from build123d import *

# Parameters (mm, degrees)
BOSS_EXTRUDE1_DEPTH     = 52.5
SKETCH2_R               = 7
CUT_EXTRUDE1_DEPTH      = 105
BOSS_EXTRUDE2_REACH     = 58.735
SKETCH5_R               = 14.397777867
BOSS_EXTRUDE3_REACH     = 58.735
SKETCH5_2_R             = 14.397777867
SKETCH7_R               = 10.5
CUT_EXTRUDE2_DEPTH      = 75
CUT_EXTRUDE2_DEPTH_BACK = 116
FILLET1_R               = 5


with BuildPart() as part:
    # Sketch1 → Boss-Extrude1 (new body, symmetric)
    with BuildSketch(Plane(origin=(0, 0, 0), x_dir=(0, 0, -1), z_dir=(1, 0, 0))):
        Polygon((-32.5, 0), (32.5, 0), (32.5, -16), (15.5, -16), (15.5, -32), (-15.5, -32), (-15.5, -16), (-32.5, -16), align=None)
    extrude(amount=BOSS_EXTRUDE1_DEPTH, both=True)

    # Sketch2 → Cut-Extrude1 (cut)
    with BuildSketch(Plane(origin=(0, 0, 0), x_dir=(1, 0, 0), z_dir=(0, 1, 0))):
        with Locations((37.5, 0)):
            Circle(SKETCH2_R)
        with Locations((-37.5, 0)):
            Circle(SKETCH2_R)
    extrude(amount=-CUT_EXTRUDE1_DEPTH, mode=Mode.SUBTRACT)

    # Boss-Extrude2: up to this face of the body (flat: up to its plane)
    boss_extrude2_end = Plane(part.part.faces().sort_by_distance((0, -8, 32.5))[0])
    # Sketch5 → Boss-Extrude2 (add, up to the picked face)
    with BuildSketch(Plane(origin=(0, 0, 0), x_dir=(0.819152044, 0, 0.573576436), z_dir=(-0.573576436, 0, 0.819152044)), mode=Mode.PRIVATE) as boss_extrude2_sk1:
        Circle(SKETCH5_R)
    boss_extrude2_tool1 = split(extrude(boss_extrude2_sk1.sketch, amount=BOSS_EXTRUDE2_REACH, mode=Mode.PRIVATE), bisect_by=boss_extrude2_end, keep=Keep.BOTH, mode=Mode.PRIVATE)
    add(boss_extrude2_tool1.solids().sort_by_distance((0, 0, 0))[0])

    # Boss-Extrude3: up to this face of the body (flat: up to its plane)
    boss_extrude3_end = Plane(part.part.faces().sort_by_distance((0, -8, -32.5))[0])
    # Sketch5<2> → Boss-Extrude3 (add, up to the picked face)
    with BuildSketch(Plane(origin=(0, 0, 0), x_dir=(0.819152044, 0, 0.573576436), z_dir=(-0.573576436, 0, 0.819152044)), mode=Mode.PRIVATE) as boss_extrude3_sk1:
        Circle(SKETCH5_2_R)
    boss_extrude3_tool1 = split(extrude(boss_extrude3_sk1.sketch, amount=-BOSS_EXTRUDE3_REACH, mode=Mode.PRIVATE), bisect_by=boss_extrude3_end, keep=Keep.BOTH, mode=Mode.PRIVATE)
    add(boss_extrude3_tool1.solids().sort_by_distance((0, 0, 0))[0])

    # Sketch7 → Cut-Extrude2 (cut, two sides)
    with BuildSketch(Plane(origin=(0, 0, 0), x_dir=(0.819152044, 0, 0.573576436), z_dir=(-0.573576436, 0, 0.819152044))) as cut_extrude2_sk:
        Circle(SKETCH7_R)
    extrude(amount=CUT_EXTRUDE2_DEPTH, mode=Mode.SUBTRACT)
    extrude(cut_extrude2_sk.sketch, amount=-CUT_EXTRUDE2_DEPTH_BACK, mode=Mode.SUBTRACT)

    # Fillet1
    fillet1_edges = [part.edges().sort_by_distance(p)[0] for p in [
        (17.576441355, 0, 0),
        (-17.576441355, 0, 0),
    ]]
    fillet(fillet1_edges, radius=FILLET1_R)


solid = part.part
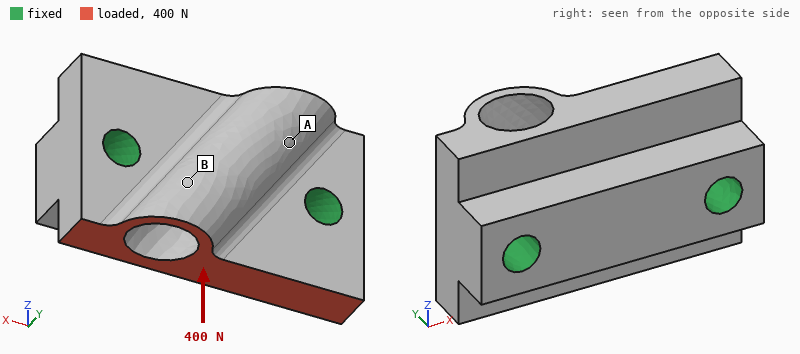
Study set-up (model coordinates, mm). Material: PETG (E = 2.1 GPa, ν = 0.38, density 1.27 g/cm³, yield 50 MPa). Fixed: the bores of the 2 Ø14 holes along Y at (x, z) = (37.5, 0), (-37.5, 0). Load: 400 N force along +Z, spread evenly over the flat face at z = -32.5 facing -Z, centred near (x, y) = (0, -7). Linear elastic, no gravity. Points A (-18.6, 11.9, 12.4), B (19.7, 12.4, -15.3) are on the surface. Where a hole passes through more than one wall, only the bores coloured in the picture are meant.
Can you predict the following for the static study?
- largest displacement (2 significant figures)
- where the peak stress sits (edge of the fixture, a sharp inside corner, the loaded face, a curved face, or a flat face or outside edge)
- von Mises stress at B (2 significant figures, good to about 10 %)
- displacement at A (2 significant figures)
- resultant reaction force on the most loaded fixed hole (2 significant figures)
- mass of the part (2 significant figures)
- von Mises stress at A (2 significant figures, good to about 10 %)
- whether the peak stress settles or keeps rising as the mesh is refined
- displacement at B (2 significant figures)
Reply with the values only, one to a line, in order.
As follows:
23 µm
a sharp inside corner
0.37 MPa
6.0 µm
210 N
190 g
0.13 MPa
keeps rising
12 µm
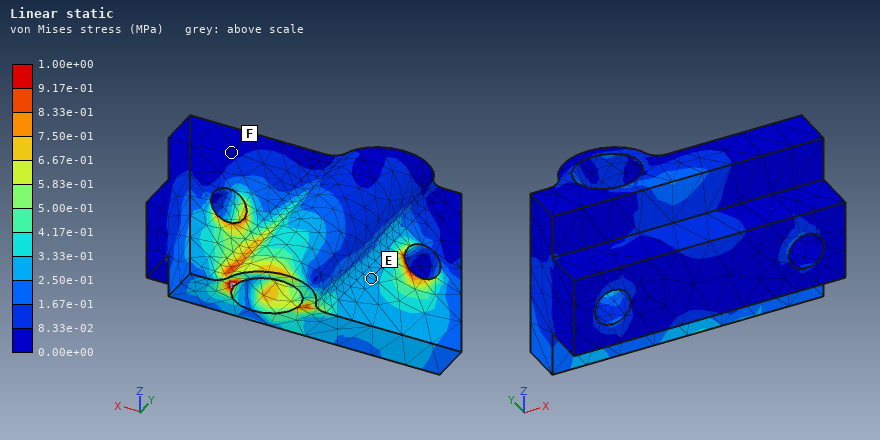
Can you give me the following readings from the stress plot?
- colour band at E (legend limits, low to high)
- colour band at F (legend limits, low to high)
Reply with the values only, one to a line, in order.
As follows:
2.50e-01 to 3.33e-01 MPa
0.00e+00 to 8.33e-02 MPa
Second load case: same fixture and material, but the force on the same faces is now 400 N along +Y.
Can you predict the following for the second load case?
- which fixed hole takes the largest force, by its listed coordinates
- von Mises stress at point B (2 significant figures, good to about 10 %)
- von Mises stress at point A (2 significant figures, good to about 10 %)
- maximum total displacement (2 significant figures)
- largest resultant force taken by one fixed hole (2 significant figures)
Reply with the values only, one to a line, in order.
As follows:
(-37.5, 0)
0.55 MPa
0.37 MPa
60 µm
220 N
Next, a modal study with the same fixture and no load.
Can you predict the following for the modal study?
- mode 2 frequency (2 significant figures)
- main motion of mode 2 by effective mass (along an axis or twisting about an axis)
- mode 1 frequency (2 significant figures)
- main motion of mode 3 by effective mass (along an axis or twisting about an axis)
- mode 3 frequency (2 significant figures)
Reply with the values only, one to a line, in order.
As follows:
3600 Hz
along Y
2800 Hz
along Z
3900 Hz
